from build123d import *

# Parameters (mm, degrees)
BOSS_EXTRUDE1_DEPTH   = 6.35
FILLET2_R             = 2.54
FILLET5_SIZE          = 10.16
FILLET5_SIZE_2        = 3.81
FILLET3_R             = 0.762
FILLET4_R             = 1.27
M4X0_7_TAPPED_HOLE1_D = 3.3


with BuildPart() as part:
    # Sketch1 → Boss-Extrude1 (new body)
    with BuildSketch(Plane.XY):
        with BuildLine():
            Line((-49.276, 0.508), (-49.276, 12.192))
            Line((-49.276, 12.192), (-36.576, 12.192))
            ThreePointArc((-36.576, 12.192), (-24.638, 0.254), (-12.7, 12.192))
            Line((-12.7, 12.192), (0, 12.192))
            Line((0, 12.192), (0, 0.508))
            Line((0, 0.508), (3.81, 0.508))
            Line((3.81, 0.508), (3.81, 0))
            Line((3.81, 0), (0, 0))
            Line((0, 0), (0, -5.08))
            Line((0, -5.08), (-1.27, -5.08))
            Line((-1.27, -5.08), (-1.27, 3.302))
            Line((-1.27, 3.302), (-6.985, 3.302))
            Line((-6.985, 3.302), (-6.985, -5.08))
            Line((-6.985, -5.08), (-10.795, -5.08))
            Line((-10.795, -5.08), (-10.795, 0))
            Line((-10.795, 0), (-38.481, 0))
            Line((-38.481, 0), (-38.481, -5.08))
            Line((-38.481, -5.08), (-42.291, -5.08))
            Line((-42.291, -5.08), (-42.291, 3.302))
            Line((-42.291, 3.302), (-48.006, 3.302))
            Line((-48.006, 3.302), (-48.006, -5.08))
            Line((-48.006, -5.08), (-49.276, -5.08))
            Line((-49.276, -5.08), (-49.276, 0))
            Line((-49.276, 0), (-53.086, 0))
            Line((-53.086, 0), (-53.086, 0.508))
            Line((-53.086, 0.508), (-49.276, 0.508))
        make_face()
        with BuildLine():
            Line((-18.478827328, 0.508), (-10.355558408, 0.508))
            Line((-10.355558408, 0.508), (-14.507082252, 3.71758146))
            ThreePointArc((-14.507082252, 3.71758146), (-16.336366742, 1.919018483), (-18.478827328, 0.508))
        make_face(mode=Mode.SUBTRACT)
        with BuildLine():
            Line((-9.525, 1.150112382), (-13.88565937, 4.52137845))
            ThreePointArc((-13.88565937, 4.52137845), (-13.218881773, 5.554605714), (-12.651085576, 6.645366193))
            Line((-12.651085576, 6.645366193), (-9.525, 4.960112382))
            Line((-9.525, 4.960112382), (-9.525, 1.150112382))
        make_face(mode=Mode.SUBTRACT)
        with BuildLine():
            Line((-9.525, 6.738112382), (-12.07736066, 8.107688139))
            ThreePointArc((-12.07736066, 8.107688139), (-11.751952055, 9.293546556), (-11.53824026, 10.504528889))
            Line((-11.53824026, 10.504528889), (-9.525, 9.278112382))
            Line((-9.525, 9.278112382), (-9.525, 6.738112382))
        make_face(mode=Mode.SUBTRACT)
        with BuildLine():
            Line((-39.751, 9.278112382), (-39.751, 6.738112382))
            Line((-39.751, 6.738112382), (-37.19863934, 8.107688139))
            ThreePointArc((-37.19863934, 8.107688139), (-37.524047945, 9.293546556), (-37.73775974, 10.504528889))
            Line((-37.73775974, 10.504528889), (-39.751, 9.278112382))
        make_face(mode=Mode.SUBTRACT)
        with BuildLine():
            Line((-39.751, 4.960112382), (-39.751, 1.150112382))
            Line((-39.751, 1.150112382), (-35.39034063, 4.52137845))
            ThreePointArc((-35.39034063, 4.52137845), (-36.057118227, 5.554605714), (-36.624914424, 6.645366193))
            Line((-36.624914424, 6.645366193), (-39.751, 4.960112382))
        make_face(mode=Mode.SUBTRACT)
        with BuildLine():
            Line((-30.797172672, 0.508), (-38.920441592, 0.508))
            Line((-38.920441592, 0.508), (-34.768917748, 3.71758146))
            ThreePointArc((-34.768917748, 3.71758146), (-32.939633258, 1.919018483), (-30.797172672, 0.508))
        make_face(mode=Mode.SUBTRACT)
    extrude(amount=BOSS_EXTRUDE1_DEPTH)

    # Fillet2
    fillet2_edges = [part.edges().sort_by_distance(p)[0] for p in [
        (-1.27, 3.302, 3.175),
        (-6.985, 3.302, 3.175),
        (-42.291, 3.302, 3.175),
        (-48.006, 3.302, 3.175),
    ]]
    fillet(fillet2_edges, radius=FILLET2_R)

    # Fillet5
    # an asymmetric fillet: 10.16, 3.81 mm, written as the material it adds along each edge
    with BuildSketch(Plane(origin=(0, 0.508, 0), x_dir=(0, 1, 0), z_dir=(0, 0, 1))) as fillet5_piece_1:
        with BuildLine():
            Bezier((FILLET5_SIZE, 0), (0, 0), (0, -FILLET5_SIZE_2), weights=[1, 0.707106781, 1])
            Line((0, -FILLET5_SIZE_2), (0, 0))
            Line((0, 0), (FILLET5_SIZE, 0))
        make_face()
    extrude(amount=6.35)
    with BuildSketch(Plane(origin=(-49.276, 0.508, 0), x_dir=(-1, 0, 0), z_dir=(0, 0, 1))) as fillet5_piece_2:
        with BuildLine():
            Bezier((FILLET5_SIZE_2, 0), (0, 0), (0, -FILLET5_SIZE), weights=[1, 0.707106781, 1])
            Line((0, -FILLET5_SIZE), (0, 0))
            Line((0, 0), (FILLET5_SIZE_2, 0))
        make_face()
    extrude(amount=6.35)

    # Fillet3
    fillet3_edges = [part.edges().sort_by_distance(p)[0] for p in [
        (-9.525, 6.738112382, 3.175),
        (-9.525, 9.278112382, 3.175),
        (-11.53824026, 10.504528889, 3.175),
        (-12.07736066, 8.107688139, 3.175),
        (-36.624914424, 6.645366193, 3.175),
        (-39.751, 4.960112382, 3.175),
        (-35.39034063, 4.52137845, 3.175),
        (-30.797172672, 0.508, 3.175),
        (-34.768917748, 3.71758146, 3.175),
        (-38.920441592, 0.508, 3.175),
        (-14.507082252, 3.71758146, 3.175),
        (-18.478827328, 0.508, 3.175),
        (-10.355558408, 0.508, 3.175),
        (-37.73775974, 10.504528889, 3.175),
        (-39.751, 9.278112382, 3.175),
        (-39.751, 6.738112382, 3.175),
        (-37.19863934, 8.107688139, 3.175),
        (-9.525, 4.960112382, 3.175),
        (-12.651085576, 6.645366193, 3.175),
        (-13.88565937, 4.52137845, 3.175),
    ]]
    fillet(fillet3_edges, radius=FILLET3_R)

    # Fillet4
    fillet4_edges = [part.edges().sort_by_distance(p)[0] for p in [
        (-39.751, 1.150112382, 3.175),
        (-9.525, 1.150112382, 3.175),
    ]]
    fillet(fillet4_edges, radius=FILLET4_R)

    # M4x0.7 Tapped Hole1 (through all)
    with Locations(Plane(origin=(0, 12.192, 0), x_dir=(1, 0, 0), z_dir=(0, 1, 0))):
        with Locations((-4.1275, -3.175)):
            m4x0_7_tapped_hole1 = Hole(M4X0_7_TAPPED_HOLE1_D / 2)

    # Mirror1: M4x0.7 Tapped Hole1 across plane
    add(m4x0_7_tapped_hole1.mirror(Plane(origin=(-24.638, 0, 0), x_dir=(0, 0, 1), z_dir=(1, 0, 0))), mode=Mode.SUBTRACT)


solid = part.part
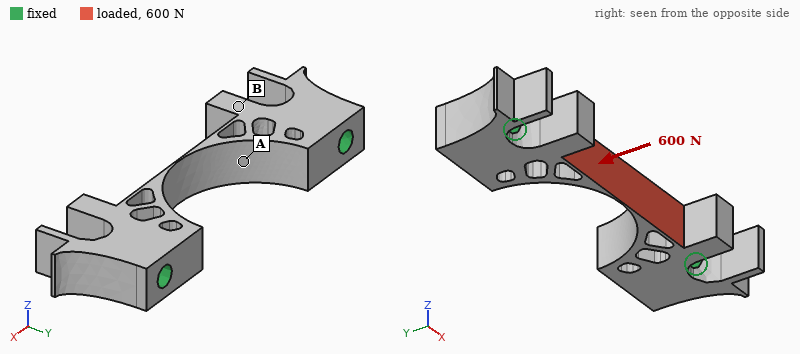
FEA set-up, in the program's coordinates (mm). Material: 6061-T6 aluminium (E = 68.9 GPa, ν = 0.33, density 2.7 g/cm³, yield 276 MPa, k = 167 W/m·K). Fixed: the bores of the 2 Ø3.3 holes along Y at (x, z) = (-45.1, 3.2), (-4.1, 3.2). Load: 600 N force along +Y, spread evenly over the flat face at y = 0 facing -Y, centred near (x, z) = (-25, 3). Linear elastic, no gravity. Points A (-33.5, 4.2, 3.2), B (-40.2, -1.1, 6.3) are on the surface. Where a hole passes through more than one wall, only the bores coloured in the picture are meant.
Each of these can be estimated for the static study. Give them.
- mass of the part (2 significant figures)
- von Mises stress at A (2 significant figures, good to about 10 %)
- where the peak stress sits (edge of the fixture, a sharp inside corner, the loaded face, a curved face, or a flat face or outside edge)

5.8 g
65 MPa
the loaded face
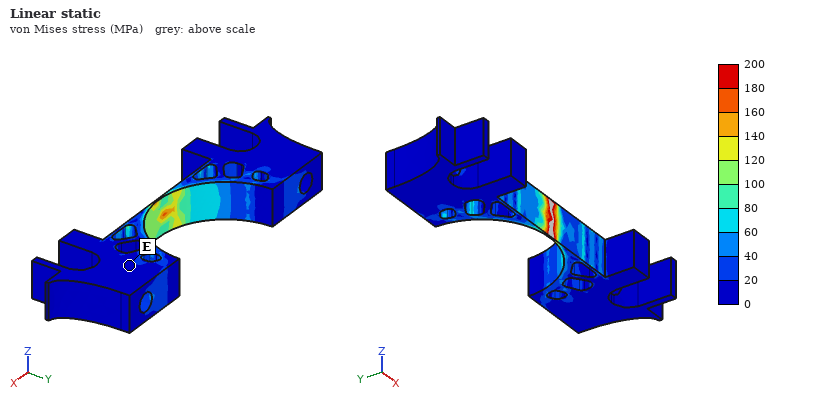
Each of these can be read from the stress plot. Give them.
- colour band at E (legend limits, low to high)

0 to 20 MPa
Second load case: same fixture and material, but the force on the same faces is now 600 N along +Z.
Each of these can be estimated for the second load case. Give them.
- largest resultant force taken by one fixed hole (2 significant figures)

300 N
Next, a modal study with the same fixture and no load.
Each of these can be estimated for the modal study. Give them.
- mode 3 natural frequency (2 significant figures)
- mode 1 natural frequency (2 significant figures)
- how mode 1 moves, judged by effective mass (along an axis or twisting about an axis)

26 kHz
21 kHz
along Z
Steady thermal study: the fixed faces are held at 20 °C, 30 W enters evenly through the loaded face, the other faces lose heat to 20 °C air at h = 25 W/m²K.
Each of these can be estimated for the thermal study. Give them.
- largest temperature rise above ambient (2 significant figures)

75 K
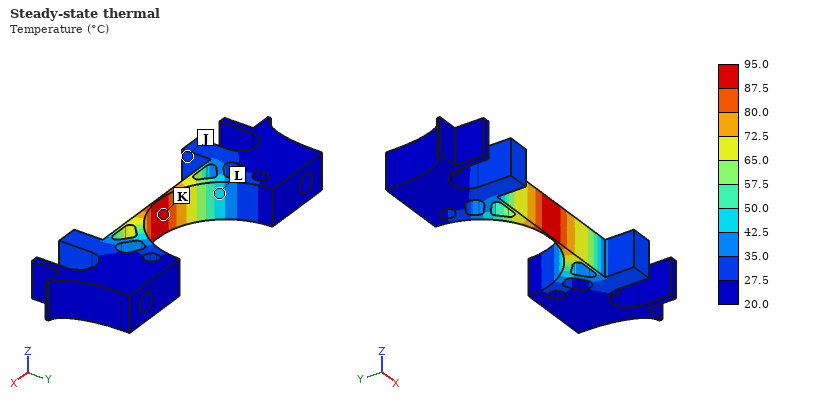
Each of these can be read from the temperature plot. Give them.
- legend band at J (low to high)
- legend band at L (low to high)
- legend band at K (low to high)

27.5 to 35.0 °C
42.5 to 50.0 °C
87.5 to 95.0 °C
